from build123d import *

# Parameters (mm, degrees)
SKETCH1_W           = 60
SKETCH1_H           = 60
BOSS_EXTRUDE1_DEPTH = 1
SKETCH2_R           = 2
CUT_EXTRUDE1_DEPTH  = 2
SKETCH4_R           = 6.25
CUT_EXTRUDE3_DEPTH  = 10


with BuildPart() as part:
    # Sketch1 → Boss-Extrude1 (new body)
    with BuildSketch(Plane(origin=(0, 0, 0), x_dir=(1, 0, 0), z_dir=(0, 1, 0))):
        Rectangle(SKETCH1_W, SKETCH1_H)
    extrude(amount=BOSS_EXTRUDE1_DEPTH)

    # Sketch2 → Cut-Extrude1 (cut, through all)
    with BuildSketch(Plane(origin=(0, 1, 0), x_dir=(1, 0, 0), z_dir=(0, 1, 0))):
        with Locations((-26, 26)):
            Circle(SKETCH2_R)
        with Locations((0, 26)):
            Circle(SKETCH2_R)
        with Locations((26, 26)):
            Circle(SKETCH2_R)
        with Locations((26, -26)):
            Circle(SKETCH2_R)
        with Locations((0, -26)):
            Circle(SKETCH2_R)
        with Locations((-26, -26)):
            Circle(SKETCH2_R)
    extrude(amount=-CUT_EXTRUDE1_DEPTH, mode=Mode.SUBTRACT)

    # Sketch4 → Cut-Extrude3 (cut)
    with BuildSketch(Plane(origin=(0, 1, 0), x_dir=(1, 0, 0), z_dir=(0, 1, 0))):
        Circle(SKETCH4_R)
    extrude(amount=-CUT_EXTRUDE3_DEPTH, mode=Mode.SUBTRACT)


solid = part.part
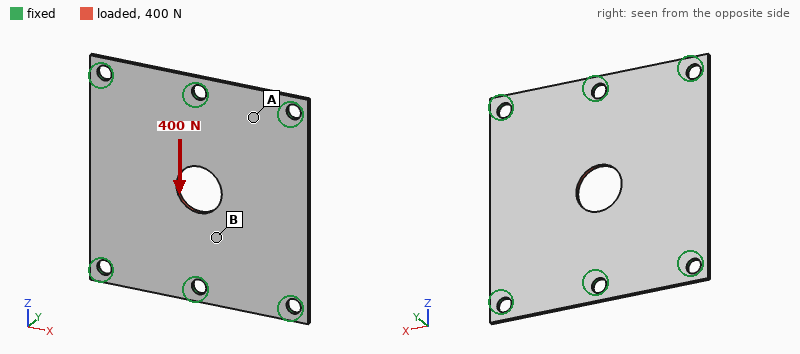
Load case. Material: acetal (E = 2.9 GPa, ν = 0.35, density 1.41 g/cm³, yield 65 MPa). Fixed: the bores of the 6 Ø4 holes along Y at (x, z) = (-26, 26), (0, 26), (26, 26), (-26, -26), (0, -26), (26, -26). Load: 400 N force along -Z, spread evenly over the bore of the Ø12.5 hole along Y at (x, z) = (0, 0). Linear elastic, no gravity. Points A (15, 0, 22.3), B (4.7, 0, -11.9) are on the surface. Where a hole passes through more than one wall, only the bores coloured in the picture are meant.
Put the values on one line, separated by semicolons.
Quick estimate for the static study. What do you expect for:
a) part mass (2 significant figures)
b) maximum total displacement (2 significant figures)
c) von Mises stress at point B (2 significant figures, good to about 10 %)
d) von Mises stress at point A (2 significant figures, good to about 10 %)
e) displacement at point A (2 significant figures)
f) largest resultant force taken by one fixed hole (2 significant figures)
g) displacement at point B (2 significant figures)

4.8 g; 67 µm; 7.8 MPa; 3.1 MPa; 21 µm; 110 N; 42 µm
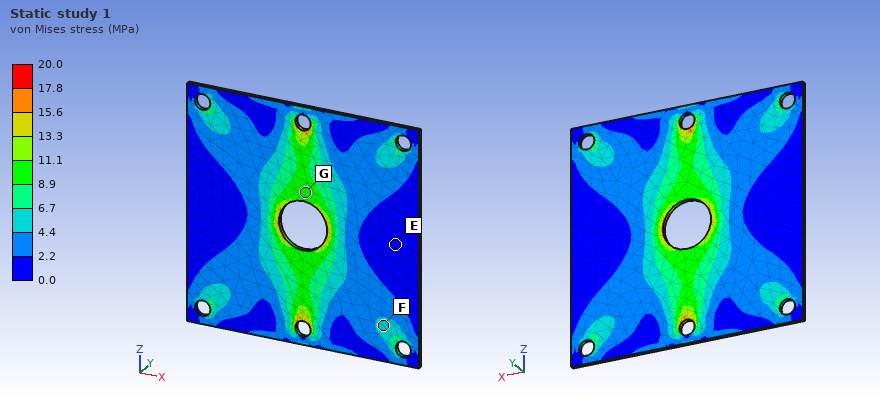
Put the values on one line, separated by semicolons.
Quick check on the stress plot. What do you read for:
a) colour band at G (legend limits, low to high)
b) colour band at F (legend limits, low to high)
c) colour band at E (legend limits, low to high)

8.9 to 11.1 MPa; 4.4 to 6.7 MPa; 0.0 to 2.2 MPa
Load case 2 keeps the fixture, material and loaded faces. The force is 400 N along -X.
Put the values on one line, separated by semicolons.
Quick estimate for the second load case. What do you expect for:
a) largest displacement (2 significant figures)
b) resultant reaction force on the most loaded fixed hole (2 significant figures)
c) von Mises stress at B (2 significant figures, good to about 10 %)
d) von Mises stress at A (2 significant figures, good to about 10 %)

0.10 mm; 87 N; 7.2 MPa; 5.3 MPa
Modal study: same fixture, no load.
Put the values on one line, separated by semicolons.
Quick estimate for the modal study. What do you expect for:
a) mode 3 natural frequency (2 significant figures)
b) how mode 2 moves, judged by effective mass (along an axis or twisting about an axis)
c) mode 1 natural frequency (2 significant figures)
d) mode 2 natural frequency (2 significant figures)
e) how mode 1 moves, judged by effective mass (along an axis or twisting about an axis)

1000 Hz; twisting about Z; 570 Hz; 670 Hz; along Y
